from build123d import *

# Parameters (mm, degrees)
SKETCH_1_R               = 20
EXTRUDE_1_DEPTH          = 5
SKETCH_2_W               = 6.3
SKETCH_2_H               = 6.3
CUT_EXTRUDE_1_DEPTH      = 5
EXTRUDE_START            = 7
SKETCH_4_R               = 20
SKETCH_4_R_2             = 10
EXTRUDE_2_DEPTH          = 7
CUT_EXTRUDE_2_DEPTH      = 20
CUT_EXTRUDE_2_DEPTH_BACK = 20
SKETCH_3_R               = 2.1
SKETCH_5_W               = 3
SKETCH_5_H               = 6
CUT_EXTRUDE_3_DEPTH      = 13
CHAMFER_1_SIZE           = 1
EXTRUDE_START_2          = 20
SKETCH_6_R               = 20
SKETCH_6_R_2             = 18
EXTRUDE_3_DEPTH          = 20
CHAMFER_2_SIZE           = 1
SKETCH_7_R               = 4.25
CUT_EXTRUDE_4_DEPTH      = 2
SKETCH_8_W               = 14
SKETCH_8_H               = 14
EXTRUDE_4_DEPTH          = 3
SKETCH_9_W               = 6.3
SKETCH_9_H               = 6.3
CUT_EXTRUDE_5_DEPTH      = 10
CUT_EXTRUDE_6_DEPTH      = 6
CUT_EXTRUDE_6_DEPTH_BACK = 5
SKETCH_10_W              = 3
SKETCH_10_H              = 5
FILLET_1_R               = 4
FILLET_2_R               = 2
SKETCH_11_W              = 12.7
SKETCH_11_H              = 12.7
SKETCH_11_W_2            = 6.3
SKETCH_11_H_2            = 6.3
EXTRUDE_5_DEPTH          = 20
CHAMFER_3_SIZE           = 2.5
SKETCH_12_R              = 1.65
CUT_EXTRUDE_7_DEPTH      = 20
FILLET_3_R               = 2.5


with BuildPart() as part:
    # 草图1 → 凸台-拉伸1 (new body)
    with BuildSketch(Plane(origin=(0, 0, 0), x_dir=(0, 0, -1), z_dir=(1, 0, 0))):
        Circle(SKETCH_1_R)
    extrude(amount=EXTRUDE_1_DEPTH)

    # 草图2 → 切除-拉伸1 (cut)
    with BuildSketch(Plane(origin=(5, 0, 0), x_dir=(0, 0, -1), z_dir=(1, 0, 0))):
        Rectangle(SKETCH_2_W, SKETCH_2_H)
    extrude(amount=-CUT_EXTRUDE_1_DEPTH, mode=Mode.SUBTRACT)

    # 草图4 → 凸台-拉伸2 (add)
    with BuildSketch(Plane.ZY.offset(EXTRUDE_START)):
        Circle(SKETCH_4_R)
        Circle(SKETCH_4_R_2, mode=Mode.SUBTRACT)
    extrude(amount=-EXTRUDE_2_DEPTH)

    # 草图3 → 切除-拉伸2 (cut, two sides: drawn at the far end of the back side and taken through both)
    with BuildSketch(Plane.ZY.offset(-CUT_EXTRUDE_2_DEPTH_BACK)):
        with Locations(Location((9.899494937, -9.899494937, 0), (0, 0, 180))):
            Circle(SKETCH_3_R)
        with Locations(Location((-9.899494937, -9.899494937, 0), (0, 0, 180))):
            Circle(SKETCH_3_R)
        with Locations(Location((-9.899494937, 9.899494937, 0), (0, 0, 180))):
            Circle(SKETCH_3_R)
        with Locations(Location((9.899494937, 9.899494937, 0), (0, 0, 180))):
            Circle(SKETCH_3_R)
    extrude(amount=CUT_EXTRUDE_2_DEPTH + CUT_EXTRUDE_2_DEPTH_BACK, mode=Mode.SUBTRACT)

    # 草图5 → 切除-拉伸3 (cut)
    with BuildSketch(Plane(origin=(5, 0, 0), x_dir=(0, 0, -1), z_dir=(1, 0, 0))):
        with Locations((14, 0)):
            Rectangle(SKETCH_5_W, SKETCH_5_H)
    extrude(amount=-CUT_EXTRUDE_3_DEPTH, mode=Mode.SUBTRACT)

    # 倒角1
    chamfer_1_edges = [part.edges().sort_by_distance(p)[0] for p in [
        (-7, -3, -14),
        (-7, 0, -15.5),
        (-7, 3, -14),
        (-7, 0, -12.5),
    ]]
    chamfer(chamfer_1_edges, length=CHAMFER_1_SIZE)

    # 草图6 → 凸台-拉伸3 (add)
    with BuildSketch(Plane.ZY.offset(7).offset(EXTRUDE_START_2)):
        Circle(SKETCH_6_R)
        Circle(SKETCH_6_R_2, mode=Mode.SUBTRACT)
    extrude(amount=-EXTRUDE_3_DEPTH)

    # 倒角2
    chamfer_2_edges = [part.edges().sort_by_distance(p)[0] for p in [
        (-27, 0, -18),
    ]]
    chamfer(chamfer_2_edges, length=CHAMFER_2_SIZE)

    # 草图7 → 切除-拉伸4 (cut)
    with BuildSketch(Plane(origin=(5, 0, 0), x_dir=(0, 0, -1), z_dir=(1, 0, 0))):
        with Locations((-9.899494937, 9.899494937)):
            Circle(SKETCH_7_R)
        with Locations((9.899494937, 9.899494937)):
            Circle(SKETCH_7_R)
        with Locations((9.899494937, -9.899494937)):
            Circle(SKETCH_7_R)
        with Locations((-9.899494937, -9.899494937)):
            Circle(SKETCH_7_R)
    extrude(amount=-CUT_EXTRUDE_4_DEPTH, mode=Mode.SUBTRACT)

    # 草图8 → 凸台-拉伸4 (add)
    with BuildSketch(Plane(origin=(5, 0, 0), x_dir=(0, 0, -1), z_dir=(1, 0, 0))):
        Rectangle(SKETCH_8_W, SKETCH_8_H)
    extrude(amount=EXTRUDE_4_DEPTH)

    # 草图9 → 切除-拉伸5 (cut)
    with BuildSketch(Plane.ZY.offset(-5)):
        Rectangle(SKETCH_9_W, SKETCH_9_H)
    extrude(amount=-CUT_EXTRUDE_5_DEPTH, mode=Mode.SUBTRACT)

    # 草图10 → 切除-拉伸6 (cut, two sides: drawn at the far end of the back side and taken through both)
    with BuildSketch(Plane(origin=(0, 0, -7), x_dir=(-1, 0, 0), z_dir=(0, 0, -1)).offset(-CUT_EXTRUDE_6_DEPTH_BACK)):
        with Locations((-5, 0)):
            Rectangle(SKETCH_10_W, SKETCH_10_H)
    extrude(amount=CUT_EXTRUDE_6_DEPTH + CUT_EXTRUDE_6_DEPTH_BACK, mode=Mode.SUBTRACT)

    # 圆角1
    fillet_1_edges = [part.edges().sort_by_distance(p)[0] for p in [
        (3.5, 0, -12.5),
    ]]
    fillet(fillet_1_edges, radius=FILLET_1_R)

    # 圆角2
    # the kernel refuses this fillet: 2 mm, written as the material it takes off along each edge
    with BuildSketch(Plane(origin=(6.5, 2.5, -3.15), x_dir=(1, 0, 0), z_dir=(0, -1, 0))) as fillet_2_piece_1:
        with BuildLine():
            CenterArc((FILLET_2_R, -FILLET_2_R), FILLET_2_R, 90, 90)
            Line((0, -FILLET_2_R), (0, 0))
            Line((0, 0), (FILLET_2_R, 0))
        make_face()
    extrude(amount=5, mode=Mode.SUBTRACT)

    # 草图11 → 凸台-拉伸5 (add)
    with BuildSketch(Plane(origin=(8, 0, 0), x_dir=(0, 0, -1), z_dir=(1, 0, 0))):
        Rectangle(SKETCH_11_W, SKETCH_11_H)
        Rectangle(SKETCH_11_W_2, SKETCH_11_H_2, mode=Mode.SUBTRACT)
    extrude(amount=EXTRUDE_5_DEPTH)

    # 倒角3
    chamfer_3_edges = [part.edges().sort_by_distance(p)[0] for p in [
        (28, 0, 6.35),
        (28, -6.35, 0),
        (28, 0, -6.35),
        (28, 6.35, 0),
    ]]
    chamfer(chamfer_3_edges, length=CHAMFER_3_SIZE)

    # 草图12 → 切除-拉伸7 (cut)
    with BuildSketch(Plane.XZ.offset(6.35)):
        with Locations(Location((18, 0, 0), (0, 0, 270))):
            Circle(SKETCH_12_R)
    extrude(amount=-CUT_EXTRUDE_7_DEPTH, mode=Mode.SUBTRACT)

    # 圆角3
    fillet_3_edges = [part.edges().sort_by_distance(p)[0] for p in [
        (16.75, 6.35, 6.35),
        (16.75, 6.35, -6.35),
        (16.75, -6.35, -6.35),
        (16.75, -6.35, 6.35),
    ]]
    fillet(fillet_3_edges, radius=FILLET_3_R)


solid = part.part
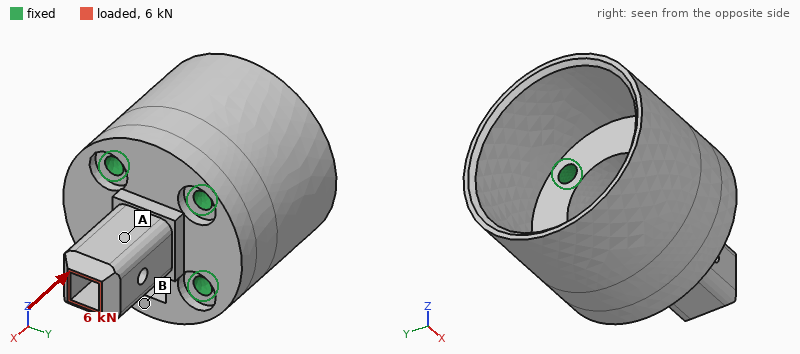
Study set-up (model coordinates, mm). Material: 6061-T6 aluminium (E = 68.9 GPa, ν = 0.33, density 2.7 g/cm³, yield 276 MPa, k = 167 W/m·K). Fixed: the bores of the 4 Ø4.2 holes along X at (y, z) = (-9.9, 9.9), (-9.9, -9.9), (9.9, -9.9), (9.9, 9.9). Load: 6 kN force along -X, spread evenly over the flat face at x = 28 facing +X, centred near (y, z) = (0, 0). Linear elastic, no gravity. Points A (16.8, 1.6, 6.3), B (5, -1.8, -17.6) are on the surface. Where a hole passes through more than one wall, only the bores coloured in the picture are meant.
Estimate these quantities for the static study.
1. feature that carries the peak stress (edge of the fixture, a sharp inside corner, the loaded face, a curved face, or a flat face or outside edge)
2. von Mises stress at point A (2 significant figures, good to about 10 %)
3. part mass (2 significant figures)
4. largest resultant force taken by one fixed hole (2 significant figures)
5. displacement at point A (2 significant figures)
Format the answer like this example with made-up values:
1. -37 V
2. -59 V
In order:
1. the loaded face
2. 52 MPa
3. 50 g
4. 1.7 kN
5. 17 µm
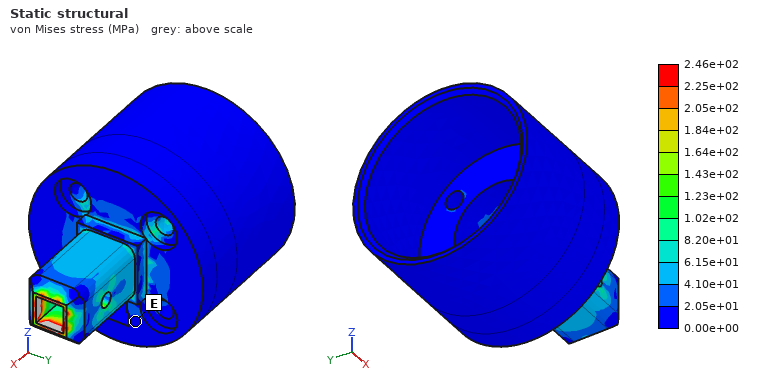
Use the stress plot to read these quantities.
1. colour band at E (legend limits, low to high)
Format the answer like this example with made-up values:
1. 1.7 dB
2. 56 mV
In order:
1. 0.00e+00 to 2.05e+01 MPa
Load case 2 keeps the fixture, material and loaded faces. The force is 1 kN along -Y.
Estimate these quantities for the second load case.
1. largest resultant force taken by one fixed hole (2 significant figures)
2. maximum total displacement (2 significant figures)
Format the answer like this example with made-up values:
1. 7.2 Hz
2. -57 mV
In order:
1. 850 N
2. 70 µm
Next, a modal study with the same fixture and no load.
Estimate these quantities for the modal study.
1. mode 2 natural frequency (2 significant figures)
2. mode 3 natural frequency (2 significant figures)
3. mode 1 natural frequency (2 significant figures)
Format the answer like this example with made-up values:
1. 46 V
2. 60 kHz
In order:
1. 13 kHz
2. 14 kHz
3. 12 kHz
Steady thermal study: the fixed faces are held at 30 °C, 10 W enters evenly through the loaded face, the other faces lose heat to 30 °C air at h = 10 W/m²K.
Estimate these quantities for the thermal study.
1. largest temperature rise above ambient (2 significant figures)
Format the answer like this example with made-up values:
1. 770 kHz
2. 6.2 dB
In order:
1. 17 K
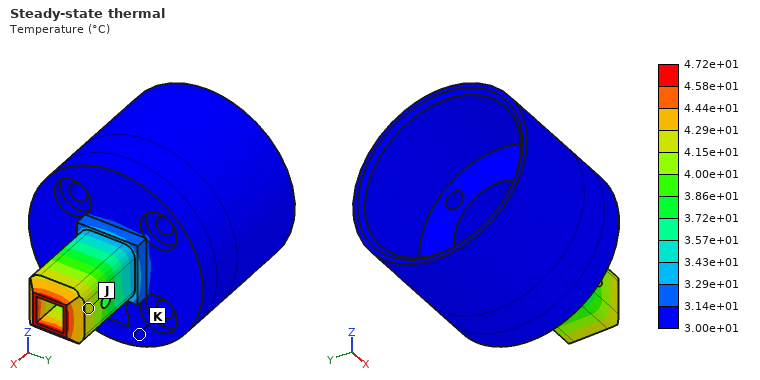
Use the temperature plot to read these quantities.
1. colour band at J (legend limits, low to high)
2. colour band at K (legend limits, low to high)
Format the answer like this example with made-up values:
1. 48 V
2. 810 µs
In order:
1. 4.15e+01 to 4.29e+01 °C
2. 3.00e+01 to 3.14e+01 °C
